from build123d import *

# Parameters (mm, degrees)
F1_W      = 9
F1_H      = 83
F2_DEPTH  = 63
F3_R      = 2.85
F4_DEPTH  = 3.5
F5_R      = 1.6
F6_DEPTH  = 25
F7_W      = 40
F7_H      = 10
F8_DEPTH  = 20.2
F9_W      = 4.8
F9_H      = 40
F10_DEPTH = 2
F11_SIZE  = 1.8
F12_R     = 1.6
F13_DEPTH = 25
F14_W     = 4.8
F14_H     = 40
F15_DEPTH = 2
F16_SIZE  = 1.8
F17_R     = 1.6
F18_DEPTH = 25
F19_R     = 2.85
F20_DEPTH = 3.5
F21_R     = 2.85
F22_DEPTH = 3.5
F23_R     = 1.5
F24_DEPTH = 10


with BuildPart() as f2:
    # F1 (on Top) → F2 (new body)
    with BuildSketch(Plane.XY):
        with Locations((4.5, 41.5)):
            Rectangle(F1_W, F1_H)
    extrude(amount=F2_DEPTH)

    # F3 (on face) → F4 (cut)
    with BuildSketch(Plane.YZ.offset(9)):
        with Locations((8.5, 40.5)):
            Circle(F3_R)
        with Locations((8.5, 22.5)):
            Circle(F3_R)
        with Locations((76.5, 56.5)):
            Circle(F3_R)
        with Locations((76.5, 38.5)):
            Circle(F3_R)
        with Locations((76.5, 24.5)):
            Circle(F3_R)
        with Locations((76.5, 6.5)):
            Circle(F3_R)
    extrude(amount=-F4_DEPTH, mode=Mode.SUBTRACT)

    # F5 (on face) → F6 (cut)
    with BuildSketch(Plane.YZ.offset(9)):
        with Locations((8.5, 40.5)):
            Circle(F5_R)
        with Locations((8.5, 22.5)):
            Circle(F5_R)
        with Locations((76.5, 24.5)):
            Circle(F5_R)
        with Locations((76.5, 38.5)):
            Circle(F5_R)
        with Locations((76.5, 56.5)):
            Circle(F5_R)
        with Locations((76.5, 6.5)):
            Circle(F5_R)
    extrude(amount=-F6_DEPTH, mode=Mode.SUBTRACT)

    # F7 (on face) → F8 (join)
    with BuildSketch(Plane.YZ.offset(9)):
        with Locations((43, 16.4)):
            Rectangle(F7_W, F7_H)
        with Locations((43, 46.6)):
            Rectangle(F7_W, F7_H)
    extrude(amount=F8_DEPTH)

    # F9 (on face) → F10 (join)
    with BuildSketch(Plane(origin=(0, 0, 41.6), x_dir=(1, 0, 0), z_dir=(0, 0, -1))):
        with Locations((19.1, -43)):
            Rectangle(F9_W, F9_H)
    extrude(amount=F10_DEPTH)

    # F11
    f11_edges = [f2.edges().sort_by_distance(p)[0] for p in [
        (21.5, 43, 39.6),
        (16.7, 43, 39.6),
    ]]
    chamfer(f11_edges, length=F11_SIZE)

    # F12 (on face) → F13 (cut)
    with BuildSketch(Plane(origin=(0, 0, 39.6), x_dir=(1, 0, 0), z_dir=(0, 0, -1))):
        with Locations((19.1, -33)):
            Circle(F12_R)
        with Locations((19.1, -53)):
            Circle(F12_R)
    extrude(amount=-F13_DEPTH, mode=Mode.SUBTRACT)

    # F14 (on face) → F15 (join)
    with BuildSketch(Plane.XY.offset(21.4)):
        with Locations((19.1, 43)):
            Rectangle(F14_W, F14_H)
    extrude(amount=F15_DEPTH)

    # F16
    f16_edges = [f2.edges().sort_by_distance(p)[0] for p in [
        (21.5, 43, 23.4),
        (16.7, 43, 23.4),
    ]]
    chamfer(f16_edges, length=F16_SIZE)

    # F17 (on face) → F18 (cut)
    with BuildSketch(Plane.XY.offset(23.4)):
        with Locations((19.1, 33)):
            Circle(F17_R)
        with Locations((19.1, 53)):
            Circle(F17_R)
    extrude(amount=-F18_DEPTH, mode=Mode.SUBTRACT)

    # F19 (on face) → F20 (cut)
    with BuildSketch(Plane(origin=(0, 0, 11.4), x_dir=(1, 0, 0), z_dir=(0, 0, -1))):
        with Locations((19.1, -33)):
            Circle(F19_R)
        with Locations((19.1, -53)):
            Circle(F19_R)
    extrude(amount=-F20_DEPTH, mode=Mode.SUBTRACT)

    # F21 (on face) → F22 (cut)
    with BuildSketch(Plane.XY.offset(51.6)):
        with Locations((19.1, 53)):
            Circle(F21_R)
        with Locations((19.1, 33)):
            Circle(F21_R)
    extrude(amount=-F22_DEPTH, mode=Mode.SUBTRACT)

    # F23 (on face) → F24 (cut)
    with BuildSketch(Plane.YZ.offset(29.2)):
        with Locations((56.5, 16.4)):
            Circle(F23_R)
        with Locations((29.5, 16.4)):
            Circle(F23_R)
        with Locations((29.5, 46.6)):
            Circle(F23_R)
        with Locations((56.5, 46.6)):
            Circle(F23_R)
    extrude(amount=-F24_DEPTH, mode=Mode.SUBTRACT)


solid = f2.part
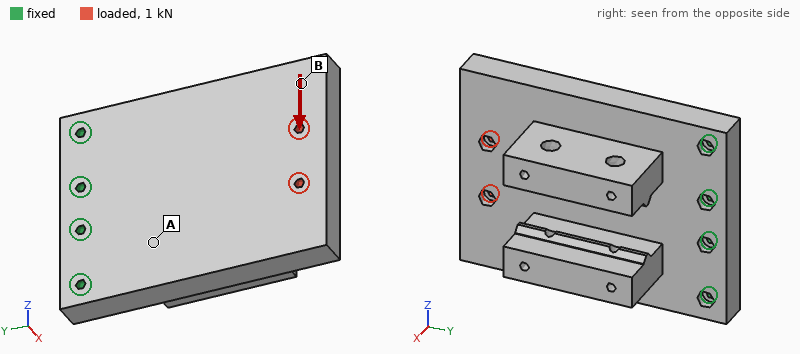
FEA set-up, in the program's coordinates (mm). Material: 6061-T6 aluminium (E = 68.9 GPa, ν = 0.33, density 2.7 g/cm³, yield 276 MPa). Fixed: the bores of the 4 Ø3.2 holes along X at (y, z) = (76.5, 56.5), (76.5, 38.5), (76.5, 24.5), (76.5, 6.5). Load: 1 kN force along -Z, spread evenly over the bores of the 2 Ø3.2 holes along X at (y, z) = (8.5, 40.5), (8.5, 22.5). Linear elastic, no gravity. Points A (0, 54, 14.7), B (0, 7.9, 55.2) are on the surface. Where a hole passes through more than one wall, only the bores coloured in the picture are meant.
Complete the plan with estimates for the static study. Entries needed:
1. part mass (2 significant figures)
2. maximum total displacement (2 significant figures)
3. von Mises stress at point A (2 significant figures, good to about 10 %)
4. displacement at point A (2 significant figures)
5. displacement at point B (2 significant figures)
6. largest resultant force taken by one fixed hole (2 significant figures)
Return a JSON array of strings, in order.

["170 g", "25 µm", "7.3 MPa", "6.0 µm", "21 µm", "1.3 kN"]
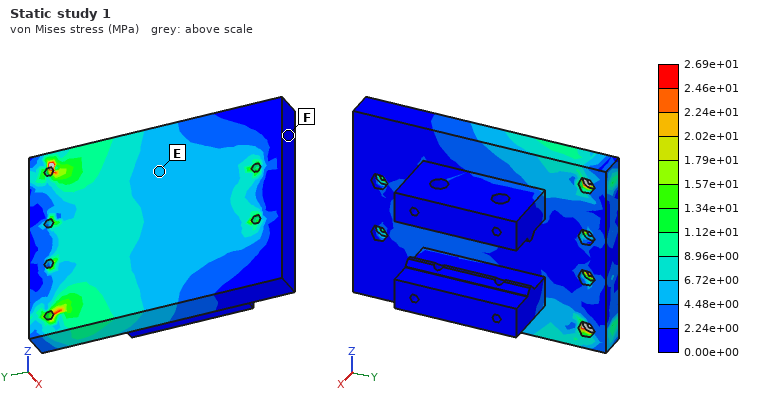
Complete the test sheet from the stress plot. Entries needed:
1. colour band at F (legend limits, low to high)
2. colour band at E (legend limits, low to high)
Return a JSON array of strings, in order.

["0.00e+00 to 2.24e+00 MPa", "4.48e+00 to 6.72e+00 MPa"]
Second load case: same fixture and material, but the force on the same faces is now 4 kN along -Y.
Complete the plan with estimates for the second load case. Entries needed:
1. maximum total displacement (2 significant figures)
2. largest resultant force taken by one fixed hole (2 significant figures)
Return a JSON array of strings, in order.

["57 µm", "1.1 kN"]
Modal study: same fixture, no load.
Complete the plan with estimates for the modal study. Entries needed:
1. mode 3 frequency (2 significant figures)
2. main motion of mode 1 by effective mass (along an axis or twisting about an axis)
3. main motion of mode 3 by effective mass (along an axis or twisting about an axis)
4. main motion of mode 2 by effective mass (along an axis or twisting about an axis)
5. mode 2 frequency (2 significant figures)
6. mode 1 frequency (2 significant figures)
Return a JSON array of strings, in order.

["5100 Hz", "along X", "along Z", "twisting about Y", "3000 Hz", "990 Hz"]
